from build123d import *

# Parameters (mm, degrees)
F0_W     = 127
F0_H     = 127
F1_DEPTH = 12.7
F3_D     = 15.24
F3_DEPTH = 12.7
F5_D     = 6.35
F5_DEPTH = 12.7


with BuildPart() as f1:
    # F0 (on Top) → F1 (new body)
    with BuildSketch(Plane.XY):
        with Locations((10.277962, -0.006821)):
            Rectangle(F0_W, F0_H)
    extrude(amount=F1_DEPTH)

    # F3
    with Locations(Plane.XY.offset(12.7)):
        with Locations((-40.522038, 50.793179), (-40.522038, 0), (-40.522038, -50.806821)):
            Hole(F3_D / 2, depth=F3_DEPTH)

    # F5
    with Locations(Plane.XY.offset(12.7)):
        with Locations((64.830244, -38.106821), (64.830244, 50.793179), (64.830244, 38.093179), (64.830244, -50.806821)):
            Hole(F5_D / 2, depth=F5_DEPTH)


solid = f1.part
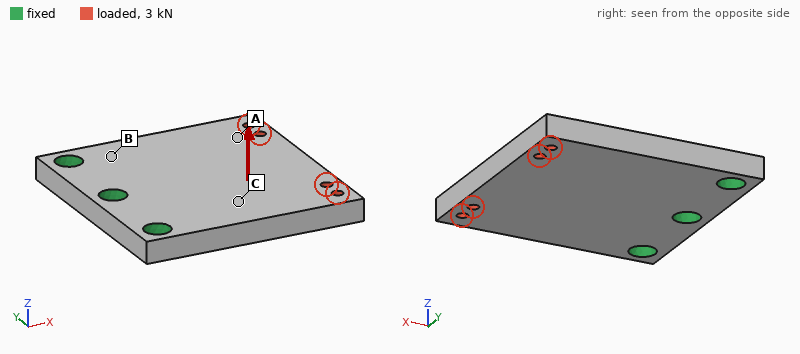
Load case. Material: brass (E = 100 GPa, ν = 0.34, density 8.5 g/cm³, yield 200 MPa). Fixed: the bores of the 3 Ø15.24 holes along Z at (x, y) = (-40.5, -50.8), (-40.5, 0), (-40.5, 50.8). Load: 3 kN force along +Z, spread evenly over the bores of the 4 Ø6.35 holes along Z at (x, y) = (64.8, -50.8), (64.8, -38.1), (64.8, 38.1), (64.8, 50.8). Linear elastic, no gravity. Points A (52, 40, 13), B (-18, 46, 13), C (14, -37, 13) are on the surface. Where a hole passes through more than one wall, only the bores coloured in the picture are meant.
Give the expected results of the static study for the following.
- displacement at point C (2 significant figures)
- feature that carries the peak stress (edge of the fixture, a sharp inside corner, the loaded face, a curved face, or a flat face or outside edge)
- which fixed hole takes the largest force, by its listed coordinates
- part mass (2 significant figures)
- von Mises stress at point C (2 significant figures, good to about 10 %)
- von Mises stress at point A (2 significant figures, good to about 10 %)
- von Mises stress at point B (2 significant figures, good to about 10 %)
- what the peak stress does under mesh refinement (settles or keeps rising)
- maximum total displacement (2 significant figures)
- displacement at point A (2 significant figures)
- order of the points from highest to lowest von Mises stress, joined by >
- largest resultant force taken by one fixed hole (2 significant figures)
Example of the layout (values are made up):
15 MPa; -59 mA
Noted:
0.15 mm; edge of the fixture; (-40.5, 0); 1.7 kg; 43 MPa; 16 MPa; 70 MPa; keeps rising; 0.54 mm; 0.39 mm; B > C > A; 1.9 kN
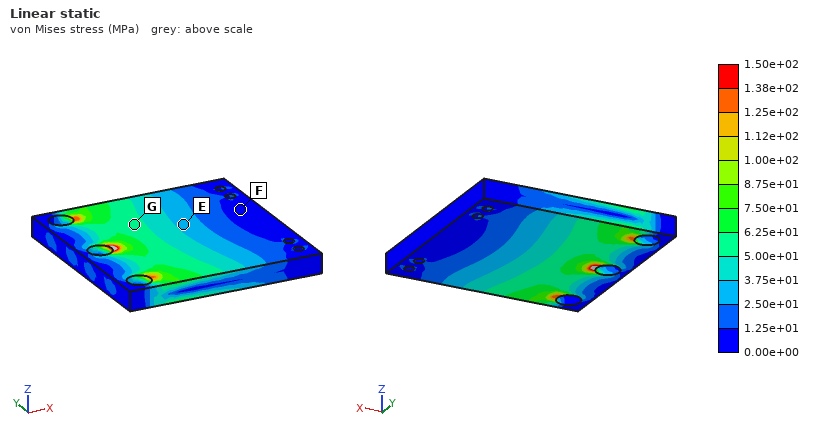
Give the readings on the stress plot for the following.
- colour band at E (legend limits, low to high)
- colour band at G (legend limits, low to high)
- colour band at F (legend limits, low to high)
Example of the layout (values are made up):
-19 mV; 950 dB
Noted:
2.50e+01 to 3.75e+01 MPa; 5.00e+01 to 6.25e+01 MPa; 0.00e+00 to 1.25e+01 MPa
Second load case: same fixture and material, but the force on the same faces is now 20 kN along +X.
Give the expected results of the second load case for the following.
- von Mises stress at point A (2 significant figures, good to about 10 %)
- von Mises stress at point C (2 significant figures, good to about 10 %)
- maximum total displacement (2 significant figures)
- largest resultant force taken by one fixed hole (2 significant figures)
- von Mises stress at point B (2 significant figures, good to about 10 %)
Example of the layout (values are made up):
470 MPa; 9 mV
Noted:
25 MPa; 13 MPa; 20 µm; 7.0 kN; 15 MPa
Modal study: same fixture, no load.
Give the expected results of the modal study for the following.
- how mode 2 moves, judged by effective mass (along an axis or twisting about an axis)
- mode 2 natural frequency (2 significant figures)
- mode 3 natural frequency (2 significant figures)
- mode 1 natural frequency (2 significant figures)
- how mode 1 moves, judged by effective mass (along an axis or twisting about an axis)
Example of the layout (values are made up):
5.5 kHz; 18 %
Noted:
twisting about X; 1300 Hz; 3200 Hz; 590 Hz; along Z
